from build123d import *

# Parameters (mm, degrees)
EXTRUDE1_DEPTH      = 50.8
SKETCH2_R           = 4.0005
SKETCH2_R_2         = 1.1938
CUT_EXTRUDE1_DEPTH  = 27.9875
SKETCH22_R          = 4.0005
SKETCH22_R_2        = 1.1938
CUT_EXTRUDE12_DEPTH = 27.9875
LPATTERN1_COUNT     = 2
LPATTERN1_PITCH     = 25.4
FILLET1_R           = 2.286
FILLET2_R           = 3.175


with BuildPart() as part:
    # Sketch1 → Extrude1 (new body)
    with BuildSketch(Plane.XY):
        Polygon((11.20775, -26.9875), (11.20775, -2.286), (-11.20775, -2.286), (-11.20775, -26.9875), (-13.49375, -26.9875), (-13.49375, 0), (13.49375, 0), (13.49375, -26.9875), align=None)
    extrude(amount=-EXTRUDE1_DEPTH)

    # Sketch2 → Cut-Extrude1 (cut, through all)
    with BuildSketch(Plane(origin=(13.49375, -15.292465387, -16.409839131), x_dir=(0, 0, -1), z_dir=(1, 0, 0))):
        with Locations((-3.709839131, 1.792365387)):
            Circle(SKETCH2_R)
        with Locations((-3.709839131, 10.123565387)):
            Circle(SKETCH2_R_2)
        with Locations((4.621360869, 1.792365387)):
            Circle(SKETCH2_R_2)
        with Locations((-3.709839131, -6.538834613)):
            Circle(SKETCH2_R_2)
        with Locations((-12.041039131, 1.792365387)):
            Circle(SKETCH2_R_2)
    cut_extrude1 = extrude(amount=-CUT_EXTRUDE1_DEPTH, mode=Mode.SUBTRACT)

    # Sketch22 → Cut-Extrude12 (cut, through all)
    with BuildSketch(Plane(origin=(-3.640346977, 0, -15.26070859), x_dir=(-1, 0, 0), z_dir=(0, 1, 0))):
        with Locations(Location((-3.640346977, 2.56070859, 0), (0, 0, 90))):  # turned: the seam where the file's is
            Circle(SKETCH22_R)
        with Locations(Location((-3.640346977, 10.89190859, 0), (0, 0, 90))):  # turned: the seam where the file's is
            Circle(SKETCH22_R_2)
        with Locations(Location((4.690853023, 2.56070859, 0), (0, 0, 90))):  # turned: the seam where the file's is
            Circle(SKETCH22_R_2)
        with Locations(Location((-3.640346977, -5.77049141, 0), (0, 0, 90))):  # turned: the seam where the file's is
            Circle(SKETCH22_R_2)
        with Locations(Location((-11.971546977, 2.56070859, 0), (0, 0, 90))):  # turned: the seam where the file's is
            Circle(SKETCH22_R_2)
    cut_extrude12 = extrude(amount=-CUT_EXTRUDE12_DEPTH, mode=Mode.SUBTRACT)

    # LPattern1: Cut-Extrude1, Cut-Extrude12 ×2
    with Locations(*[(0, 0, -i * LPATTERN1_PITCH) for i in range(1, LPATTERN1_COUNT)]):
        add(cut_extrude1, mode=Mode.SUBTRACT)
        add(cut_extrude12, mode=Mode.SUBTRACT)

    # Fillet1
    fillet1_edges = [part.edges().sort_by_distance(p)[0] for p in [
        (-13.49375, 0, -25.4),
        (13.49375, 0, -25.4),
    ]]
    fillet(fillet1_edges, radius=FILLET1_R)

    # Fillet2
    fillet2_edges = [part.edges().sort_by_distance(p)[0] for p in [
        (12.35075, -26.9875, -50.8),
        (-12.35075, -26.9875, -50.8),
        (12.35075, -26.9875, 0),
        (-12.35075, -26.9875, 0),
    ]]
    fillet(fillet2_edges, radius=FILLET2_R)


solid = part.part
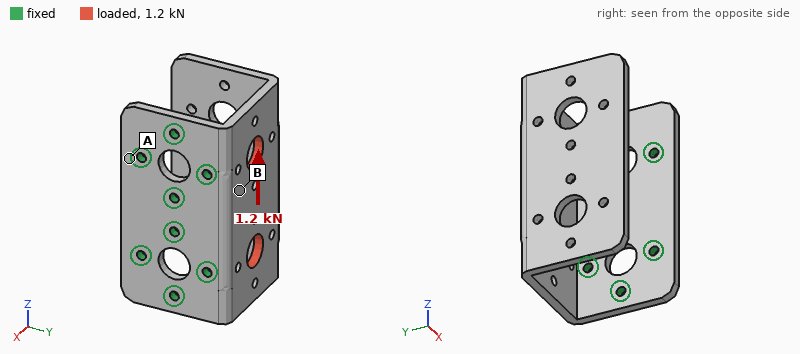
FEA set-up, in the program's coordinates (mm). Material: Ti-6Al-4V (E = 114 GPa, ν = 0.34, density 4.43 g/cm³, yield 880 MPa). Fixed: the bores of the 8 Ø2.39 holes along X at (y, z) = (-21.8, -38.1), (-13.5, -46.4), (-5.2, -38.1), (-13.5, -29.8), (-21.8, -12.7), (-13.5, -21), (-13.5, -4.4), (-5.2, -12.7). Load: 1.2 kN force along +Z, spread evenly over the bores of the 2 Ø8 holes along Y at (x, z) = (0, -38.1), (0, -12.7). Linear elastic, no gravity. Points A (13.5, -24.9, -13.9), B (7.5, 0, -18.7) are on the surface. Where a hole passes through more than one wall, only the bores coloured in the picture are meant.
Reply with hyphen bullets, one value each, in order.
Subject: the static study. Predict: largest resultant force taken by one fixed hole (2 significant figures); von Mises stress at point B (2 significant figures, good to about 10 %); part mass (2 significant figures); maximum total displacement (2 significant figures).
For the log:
- 730 N
- 18 MPa
- 35 g
- 65 µm
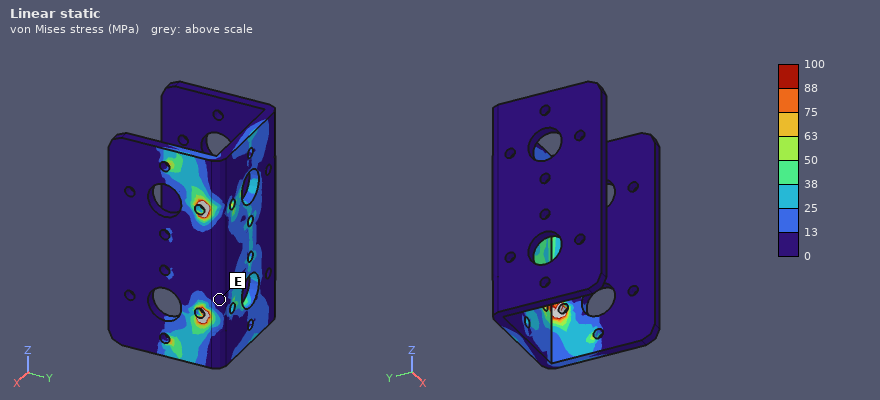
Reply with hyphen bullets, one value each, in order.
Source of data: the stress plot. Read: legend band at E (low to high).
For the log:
- 0 to 13 MPa
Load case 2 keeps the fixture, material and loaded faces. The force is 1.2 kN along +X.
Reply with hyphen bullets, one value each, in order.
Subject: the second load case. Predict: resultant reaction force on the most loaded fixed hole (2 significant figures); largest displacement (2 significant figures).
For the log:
- 660 N
- 77 µm
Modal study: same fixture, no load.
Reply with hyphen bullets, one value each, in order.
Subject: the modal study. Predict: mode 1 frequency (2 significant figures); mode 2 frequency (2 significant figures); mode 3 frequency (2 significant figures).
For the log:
- 860 Hz
- 1500 Hz
- 2400 Hz
